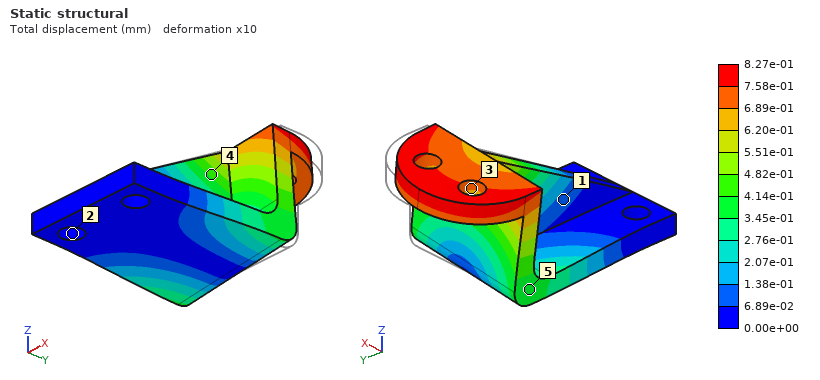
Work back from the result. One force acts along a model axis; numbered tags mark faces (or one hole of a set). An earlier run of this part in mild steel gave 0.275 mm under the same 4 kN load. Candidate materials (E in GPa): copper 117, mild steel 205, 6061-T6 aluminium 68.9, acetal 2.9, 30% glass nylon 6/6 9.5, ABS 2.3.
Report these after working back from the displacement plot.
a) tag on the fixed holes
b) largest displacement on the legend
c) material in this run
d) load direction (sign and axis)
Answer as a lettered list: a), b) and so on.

a) 2
b) 8.27e-01 mm
c) 6061-T6 aluminium
d) -X
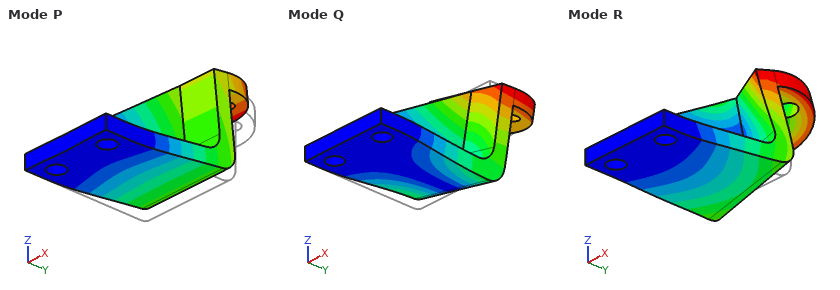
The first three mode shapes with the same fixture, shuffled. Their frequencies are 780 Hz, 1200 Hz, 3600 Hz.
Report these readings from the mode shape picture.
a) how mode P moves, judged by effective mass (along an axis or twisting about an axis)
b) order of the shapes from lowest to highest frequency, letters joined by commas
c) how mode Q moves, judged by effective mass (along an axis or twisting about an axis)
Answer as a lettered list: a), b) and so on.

a) along Z
b) P, Q, R
c) along X
